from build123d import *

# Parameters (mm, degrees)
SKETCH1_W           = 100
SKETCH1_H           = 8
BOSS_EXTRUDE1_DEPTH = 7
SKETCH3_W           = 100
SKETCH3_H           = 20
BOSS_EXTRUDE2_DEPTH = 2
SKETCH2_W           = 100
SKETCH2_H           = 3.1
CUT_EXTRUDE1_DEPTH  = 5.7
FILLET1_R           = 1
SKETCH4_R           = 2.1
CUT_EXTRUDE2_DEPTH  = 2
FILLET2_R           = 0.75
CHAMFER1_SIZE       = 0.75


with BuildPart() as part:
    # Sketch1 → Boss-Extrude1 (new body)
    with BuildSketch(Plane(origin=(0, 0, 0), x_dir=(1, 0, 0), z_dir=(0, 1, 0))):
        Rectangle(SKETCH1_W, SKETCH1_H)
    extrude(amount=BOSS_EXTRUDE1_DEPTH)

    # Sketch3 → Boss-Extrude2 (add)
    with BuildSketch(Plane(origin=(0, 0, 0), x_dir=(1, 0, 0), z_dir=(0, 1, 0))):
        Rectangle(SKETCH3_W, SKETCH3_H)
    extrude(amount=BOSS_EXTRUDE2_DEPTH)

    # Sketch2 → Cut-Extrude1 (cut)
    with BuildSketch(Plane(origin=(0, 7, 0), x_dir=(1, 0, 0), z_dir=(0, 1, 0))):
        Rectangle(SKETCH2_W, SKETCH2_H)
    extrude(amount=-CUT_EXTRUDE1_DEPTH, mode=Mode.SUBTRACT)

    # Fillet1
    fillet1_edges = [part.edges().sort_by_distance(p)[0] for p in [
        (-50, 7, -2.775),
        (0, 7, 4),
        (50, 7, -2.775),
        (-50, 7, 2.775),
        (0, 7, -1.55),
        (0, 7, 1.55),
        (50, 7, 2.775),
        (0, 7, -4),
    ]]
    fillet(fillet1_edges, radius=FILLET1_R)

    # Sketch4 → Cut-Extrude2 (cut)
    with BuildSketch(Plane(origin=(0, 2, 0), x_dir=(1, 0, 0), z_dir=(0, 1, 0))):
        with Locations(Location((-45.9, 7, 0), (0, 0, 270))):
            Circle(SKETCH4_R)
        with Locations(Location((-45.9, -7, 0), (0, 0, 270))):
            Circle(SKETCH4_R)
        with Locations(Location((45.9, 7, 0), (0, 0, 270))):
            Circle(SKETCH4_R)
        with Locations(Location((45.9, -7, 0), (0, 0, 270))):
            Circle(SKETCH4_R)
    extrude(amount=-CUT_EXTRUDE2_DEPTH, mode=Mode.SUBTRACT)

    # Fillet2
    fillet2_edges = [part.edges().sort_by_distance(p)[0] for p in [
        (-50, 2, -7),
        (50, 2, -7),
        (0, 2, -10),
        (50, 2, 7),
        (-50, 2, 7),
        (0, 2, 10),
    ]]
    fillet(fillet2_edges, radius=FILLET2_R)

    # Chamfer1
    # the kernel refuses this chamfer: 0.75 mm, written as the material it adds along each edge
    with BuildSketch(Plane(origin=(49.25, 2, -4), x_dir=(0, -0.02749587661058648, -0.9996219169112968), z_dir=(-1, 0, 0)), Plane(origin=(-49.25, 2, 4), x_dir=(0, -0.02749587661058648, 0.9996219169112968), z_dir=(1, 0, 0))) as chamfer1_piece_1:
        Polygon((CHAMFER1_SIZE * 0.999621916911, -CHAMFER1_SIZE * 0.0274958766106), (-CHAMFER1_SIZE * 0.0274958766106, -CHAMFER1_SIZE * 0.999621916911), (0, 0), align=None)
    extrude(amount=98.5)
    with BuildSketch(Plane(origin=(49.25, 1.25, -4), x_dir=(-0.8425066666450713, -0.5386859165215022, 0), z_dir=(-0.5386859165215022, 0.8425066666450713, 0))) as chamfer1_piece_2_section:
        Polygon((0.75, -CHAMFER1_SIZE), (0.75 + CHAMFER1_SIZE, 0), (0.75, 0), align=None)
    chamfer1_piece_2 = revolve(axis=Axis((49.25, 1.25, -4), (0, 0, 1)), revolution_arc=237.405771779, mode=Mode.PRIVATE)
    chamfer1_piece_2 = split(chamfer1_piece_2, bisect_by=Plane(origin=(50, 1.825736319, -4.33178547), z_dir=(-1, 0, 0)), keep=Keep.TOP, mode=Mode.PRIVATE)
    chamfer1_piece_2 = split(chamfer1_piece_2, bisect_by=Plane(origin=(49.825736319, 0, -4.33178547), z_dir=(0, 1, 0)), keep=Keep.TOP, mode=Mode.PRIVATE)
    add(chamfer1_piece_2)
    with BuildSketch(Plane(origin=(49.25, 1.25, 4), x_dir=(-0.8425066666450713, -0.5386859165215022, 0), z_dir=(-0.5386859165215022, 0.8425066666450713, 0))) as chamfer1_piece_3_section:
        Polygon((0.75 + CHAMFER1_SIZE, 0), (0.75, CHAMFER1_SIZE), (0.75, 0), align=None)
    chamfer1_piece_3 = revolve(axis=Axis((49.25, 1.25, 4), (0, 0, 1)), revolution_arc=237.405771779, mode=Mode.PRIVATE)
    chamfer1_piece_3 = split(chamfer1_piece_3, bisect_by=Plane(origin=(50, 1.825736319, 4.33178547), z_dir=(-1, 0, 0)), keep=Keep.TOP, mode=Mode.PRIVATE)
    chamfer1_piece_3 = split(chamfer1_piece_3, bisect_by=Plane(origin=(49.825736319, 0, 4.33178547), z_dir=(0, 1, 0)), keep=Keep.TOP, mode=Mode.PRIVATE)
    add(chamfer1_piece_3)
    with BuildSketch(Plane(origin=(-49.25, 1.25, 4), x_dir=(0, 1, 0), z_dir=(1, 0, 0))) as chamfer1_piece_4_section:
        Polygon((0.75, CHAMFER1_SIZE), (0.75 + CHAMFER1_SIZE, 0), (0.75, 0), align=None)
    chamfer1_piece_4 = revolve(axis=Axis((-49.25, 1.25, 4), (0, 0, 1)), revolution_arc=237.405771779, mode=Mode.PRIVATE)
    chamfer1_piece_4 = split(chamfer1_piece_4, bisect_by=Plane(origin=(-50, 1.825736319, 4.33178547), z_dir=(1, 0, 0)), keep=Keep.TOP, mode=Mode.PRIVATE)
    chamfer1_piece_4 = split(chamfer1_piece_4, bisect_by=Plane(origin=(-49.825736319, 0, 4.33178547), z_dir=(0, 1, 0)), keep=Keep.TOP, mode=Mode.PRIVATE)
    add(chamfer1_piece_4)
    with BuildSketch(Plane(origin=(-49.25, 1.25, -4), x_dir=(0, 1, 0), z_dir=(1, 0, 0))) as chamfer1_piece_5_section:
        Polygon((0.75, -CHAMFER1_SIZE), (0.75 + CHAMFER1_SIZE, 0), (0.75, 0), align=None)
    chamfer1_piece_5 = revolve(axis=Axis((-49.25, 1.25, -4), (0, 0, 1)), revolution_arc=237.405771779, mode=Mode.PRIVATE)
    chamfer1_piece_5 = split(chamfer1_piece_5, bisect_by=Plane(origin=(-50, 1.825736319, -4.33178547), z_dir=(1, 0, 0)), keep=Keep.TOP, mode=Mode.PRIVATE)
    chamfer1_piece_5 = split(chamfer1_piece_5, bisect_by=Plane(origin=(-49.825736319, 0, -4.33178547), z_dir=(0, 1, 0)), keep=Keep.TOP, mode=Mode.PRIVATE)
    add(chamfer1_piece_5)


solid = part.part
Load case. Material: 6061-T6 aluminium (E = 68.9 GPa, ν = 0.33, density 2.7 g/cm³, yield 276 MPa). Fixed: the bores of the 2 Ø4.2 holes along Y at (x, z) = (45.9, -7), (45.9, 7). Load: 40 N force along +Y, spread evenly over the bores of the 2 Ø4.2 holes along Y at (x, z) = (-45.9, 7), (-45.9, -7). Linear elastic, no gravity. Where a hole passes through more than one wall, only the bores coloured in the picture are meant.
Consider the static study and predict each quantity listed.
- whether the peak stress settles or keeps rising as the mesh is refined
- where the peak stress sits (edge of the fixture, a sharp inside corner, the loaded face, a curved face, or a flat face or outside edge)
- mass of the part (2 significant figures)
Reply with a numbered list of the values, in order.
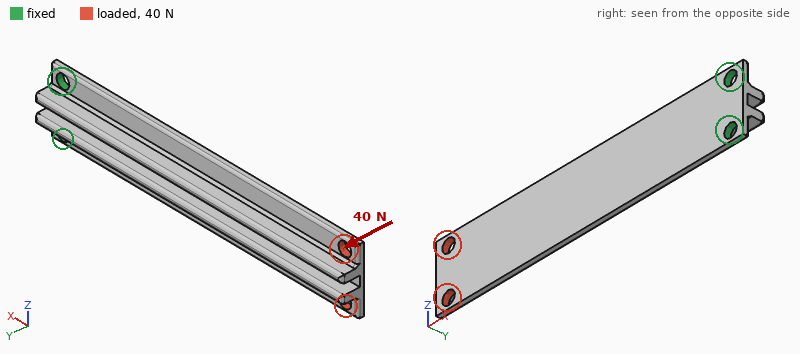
1. keeps rising
2. edge of the fixture
3. 16 g
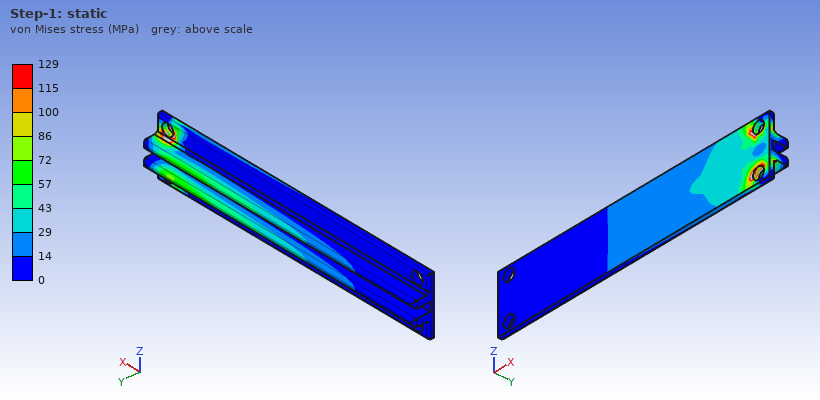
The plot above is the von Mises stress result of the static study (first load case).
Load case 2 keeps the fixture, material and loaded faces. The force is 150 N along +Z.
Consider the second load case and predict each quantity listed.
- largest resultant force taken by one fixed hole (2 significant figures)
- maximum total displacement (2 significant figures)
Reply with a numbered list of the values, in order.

1. 950 N
2. 0.41 mm
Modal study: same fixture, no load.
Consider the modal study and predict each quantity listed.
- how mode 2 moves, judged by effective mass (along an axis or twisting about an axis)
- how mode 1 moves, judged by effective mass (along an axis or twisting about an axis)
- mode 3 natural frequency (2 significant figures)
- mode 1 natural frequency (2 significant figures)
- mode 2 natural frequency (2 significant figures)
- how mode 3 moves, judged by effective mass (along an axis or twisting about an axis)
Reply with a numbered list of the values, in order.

1. along Z
2. along Y
3. 2200 Hz
4. 480 Hz
5. 1500 Hz
6. twisting about X
